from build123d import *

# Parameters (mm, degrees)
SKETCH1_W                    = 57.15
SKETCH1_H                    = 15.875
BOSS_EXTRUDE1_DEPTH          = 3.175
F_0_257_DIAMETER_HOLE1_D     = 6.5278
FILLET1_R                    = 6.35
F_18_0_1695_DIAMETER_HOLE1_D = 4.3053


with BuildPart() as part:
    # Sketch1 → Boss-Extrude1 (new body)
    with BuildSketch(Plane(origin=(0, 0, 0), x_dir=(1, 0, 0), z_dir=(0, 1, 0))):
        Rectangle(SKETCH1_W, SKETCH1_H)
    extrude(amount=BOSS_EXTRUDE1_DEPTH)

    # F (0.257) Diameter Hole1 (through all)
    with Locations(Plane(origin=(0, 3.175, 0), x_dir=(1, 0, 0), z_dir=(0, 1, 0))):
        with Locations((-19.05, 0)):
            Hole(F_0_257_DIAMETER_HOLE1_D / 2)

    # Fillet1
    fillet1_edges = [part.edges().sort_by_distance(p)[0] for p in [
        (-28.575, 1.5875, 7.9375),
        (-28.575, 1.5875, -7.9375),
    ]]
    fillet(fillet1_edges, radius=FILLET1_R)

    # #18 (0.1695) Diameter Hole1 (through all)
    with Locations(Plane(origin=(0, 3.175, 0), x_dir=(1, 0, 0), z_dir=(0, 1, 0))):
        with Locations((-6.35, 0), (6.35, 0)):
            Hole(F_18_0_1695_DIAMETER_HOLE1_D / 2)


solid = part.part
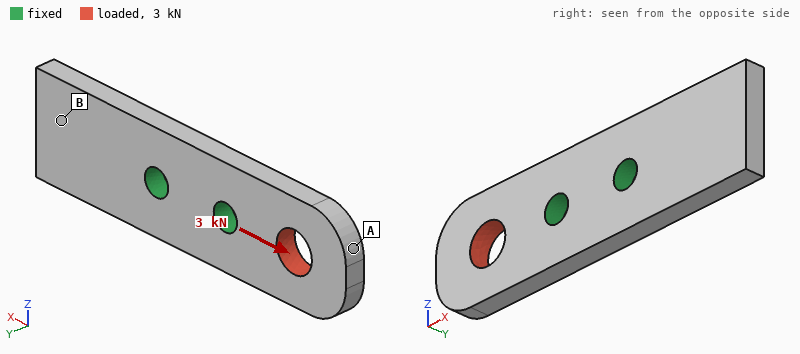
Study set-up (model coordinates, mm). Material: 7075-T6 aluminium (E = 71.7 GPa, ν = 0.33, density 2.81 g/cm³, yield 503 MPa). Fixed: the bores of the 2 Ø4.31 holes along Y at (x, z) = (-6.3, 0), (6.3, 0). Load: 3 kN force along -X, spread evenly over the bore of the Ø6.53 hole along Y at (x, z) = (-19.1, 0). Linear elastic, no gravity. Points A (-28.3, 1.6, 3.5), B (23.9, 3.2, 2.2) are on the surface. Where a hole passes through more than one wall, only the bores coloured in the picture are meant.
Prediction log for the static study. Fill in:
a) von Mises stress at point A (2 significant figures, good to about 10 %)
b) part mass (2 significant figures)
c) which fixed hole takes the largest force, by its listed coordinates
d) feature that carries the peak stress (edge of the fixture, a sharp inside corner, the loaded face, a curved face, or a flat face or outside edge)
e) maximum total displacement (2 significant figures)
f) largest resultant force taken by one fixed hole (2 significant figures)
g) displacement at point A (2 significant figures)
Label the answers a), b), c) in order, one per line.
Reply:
a) 29 MPa
b) 7.4 g
c) (-6.3, 0)
d) the loaded face
e) 21 µm
f) 2.5 kN
g) 17 µm
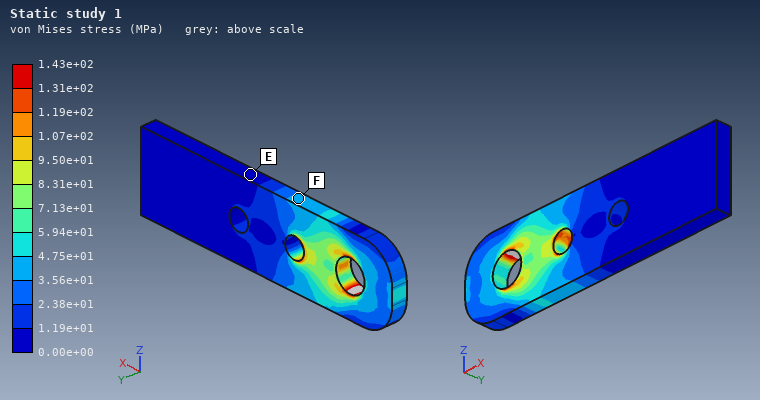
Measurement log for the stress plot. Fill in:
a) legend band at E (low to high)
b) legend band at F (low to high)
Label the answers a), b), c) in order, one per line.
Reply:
a) 0.00e+00 to 1.19e+01 MPa
b) 3.56e+01 to 4.75e+01 MPa
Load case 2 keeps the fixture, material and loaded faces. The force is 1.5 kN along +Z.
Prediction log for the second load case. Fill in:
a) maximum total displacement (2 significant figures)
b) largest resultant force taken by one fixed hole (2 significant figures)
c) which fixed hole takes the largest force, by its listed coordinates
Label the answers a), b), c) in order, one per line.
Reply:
a) 84 µm
b) 2.3 kN
c) (-6.3, 0)
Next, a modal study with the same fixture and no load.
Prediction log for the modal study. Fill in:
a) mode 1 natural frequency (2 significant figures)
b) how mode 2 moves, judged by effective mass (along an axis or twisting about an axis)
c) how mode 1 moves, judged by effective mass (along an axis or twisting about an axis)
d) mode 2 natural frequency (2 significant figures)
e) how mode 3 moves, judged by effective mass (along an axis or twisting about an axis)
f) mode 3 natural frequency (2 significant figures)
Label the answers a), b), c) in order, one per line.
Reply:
a) 5600 Hz
b) along Y
c) along Y
d) 6100 Hz
e) twisting about X
f) 14 kHz
